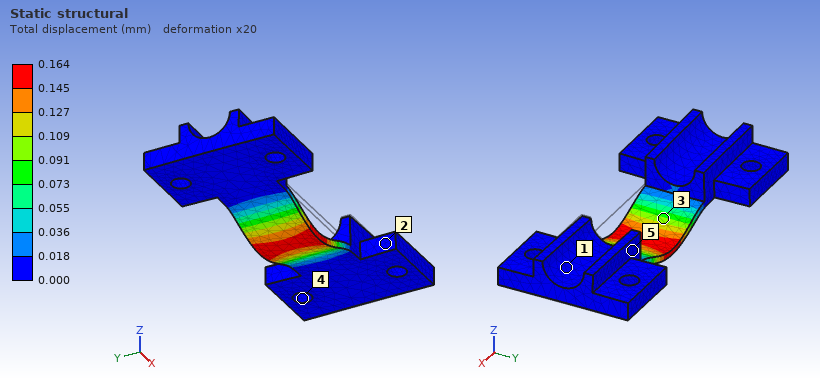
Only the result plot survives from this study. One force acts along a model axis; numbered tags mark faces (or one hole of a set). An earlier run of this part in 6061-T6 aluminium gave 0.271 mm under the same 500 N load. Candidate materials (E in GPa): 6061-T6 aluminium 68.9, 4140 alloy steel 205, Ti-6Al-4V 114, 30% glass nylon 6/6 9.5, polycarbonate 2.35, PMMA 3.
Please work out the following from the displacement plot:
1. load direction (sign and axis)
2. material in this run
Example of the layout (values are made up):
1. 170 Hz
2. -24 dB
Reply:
1. -Z
2. Ti-6Al-4V
